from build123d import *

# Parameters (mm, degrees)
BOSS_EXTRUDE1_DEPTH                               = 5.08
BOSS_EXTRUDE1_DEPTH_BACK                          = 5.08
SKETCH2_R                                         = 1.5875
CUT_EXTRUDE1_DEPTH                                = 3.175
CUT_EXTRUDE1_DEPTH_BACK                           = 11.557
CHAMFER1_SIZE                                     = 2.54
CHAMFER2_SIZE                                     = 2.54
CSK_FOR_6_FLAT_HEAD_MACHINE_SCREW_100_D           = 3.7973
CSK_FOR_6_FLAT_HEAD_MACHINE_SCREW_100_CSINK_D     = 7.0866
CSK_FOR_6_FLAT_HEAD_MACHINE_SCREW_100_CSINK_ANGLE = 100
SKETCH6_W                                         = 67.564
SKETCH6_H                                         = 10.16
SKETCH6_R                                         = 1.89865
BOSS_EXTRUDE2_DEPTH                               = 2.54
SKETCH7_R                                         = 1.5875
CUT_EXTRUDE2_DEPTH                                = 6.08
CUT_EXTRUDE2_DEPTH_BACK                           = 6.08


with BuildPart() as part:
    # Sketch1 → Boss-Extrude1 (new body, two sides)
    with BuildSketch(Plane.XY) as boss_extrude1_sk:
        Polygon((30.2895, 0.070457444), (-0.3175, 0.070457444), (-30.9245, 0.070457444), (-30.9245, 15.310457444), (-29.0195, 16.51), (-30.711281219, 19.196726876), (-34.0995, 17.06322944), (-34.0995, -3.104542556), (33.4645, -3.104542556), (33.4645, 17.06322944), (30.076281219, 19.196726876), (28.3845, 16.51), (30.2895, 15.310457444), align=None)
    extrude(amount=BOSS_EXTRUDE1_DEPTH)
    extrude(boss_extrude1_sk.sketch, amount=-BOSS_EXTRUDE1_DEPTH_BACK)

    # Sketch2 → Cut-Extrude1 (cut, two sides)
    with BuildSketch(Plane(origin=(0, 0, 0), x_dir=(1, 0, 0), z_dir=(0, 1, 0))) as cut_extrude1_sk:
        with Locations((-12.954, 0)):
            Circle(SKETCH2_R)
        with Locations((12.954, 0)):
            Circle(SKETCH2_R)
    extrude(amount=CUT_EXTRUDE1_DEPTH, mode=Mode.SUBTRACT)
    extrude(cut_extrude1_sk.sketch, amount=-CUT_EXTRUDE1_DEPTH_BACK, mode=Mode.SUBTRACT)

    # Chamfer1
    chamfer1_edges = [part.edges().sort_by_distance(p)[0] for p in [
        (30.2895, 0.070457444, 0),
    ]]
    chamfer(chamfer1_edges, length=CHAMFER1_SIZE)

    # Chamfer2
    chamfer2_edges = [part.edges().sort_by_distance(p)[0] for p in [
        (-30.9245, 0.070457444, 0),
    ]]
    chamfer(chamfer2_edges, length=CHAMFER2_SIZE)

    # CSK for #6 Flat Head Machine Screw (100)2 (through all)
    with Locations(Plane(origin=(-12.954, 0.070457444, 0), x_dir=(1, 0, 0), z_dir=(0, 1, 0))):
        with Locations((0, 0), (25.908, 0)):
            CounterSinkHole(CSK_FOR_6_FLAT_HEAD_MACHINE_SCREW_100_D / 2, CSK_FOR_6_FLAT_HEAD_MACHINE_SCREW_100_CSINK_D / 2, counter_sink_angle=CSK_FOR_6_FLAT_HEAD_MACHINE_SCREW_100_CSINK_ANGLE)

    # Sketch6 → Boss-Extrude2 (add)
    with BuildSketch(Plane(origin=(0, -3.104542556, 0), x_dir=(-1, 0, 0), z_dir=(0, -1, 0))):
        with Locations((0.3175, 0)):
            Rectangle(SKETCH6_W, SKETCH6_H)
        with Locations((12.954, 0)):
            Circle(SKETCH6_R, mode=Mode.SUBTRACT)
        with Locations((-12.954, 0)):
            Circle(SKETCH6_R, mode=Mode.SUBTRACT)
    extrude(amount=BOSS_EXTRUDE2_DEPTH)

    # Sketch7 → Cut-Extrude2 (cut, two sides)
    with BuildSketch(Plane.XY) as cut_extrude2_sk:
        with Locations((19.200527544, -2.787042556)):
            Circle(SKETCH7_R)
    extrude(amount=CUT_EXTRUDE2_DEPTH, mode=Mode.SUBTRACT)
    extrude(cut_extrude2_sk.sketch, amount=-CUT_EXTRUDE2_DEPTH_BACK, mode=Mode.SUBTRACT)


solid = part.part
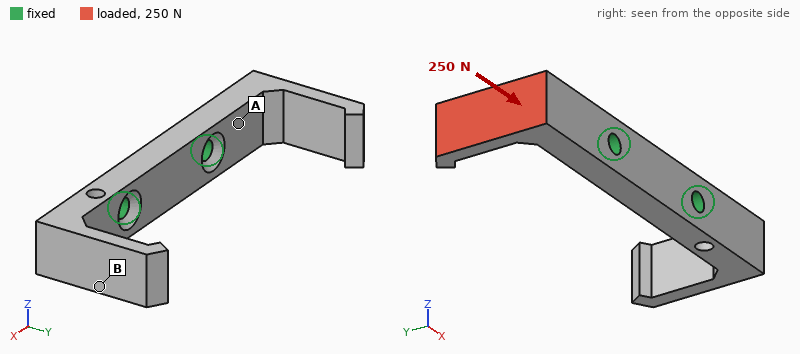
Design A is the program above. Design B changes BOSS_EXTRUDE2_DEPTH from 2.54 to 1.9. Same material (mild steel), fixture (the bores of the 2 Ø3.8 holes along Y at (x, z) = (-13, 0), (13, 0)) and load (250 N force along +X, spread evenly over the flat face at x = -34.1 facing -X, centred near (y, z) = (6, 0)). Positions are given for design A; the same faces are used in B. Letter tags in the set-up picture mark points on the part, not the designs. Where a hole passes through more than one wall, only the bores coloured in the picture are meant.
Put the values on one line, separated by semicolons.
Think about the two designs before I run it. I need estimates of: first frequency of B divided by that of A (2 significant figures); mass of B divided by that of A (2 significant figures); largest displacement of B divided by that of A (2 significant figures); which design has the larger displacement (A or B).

0.87; 0.91; 1.2; B
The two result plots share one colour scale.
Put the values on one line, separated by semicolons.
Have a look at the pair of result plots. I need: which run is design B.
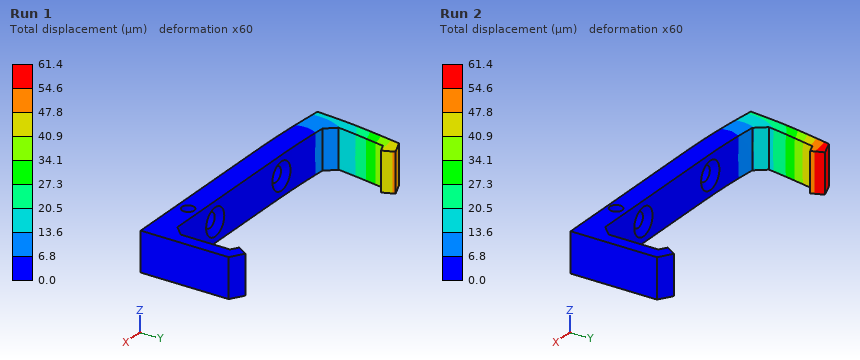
Run 2
